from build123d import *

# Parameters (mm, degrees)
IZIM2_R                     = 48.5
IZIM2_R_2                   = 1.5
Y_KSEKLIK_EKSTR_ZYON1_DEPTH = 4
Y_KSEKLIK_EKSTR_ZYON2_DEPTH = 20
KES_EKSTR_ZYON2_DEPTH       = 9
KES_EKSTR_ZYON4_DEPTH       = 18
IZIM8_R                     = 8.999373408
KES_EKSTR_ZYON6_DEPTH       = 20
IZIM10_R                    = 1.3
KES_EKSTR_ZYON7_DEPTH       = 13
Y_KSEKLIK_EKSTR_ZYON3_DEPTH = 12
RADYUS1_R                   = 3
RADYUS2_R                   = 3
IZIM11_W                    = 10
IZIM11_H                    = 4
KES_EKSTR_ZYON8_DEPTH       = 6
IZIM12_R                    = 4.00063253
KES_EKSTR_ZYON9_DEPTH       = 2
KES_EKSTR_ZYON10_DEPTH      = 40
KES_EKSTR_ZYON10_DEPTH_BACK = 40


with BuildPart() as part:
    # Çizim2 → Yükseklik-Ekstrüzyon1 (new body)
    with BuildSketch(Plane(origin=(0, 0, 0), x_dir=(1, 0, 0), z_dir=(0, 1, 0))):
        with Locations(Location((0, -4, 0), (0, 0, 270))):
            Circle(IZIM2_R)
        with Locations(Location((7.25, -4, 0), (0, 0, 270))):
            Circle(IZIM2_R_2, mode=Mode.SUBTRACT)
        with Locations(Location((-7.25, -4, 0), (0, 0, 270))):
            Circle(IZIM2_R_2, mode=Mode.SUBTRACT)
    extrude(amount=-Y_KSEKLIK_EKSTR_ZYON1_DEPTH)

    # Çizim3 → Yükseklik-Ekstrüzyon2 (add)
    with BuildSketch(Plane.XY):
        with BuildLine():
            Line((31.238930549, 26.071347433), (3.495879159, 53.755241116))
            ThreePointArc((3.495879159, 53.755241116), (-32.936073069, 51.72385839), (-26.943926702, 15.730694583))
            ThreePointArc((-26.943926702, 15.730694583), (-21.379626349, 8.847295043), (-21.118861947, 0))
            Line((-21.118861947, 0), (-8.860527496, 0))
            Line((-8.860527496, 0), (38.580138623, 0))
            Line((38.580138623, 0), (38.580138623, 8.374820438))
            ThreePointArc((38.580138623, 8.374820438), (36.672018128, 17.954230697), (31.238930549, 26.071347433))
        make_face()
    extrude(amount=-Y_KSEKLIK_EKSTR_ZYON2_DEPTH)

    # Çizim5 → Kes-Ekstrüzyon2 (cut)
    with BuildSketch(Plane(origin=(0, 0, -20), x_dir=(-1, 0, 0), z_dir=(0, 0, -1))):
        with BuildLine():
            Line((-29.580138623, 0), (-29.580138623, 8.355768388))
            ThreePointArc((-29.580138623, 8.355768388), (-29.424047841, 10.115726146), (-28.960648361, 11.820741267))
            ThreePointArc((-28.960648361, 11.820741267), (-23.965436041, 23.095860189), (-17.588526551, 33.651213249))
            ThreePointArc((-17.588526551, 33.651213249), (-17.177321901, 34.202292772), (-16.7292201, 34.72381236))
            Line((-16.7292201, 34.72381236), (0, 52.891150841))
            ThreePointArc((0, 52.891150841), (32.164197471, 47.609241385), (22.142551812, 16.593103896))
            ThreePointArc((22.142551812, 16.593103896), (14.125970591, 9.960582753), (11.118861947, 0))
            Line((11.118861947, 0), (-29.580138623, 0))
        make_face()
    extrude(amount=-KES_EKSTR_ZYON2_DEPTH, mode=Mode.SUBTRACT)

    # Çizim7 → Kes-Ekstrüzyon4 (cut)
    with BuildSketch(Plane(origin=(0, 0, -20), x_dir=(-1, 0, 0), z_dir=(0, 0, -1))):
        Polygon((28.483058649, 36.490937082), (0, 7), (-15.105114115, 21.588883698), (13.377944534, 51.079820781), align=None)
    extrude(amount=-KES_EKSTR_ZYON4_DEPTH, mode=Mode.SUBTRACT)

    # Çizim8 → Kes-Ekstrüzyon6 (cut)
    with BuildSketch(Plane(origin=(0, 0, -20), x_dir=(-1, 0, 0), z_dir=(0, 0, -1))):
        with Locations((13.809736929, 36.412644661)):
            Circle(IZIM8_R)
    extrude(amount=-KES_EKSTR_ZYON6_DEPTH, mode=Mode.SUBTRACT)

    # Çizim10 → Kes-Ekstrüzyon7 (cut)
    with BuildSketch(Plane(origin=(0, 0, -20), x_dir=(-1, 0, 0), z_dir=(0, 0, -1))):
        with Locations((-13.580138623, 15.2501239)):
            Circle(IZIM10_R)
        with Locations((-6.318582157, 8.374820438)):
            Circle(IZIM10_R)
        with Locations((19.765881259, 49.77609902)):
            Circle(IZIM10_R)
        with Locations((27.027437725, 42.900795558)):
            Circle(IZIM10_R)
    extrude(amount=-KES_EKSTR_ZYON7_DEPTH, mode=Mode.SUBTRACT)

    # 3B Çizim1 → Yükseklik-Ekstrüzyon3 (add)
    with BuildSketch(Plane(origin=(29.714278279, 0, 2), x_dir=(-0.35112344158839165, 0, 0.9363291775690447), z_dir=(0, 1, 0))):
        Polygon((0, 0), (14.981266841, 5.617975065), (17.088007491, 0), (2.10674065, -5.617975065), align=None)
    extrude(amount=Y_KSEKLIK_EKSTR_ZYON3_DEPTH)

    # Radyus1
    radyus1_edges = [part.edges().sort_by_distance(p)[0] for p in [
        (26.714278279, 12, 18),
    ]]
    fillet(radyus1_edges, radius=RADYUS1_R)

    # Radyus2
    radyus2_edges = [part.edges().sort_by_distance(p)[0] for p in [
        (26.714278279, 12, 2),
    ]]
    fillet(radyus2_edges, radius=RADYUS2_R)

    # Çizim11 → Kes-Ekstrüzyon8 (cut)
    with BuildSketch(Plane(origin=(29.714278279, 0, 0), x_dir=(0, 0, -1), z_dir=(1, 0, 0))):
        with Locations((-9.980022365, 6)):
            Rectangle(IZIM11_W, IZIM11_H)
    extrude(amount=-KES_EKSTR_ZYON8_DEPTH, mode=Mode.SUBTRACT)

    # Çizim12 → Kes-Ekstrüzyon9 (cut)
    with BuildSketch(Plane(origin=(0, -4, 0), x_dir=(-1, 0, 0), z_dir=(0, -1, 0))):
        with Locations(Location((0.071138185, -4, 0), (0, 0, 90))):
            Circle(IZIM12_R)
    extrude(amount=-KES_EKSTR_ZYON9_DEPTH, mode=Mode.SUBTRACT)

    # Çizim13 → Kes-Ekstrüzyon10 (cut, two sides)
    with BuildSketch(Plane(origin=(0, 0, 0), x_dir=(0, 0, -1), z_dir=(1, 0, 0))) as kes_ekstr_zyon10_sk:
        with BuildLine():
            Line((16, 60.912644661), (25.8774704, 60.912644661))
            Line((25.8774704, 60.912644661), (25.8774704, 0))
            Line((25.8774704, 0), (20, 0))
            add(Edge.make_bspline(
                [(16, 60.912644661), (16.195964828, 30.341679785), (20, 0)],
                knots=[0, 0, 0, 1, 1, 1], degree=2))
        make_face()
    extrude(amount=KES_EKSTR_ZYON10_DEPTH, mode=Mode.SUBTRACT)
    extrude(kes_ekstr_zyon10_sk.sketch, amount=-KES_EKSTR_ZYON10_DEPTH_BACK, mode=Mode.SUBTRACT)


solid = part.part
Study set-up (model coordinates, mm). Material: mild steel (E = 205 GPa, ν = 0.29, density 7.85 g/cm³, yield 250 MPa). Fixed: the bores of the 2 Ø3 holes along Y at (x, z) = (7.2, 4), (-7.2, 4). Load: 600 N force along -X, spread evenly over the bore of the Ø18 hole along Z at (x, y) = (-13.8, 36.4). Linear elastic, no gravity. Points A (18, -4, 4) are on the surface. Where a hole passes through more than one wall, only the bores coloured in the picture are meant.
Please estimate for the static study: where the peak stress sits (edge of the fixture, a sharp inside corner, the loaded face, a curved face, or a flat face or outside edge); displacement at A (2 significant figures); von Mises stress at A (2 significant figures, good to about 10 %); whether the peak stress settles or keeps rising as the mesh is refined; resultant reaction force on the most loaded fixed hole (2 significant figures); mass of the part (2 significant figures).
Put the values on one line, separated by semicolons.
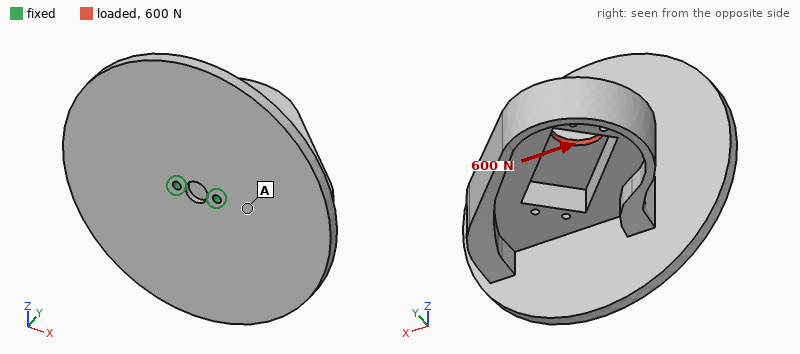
edge of the fixture; 7.1 µm; 9.8 MPa; keeps rising; 1.3 kN; 500 g
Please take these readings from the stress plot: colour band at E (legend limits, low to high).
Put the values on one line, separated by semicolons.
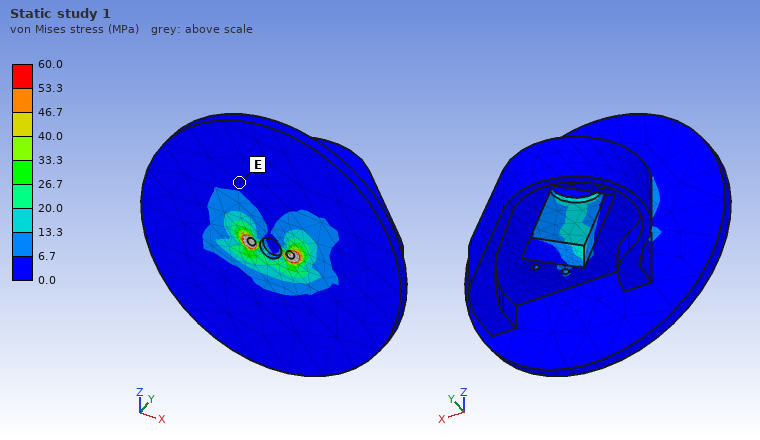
0.0 to 6.7 MPa
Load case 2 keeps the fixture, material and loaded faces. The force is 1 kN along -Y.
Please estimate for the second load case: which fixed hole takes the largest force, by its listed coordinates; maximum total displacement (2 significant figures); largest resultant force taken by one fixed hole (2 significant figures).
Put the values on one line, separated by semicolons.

(-7.2, 4); 31 µm; 1.2 kN
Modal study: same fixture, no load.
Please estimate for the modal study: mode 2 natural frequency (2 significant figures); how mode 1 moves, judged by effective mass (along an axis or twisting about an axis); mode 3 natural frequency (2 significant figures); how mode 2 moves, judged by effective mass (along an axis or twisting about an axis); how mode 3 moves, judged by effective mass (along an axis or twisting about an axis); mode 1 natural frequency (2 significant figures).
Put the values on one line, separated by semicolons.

1400 Hz; along Z; 1700 Hz; along X; along Y; 660 Hz
